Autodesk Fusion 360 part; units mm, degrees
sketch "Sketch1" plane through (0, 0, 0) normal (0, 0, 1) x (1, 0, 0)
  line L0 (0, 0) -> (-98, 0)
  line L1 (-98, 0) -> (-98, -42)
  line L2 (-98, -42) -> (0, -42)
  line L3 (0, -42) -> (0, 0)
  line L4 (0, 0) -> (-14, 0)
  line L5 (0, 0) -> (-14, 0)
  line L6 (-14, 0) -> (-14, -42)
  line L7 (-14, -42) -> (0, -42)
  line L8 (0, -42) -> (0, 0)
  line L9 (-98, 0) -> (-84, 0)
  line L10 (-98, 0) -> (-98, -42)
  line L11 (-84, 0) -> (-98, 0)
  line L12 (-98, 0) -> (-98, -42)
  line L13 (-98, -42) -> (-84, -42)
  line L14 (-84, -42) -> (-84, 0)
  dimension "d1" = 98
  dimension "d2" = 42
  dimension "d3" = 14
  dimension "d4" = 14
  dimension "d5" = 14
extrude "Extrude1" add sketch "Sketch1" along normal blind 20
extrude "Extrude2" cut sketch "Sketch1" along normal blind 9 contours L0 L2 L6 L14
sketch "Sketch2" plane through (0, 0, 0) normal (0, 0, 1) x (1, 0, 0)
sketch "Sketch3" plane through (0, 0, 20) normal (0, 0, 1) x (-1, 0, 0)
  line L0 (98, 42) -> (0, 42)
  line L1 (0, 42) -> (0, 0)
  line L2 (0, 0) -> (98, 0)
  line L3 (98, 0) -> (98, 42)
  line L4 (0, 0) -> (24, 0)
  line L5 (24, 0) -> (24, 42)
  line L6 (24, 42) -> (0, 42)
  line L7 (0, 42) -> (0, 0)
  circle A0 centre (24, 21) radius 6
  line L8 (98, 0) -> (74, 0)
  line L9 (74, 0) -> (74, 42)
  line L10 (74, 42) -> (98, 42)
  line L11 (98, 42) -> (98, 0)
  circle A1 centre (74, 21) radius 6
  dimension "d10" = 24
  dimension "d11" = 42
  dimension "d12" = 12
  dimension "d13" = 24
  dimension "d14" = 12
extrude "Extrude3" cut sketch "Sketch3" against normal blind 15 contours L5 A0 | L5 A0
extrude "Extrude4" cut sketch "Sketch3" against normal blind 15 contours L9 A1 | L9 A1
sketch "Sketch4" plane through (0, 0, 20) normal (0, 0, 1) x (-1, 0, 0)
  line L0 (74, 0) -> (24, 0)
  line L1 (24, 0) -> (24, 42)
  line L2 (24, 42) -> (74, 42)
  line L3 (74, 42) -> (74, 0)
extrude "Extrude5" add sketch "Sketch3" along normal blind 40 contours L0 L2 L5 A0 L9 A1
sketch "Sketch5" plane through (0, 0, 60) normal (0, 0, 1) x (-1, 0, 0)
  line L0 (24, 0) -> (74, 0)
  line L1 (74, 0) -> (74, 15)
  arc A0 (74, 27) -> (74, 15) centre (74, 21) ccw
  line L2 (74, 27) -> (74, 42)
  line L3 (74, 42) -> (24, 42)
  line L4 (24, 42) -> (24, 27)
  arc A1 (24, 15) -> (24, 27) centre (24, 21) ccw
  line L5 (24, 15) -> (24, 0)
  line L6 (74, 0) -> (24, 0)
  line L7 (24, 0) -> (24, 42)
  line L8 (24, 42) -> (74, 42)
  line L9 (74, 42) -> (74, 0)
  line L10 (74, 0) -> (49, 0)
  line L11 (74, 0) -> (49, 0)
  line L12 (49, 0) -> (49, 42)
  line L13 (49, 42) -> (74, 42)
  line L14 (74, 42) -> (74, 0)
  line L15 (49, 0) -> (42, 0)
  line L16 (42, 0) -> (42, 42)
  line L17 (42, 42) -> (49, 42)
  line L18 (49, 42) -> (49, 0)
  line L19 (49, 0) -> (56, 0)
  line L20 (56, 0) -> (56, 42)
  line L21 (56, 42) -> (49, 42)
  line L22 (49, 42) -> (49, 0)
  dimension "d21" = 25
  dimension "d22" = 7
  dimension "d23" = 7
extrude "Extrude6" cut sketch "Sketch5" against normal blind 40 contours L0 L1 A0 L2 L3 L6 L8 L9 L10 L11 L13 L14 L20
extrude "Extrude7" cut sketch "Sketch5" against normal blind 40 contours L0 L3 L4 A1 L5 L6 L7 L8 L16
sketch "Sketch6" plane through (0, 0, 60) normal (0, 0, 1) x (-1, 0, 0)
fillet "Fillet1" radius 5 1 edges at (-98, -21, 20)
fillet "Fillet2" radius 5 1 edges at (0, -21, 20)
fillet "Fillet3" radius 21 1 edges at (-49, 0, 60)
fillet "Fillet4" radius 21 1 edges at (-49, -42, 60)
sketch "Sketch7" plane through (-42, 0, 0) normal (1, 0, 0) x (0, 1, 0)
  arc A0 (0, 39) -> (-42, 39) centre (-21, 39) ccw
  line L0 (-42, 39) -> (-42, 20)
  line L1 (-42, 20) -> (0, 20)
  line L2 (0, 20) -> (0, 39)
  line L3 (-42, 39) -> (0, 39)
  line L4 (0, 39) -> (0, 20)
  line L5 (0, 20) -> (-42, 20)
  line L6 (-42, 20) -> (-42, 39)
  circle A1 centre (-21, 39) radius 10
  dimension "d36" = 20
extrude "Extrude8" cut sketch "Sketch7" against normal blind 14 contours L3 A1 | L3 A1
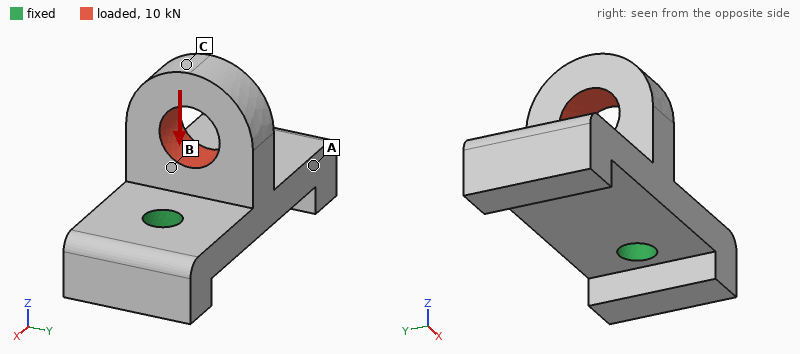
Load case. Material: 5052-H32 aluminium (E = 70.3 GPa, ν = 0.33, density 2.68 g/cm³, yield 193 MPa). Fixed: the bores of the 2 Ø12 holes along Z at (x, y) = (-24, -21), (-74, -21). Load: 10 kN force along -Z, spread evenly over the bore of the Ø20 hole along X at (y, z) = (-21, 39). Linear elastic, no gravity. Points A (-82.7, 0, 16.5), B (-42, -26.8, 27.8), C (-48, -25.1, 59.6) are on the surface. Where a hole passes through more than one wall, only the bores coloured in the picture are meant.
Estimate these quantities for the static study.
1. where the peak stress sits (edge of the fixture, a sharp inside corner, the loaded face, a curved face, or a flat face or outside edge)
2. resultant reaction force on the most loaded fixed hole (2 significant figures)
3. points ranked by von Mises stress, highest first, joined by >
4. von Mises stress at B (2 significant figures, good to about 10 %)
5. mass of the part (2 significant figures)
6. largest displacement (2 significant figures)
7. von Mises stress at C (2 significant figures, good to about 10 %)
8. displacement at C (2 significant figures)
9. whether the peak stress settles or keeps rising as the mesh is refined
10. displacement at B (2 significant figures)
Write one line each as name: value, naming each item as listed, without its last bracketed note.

where the peak stress sits: edge of the fixture
resultant reaction force on the most loaded fixed hole: 5.1 kN
points ranked by von Mises stress, highest first, joined by >: B > C > A
von Mises stress at B: 30 MPa
mass of the part: 190 g
largest displacement: 37 µm
von Mises stress at C: 21 MPa
displacement at C: 35 µm
whether the peak stress settles or keeps rising as the mesh is refined: keeps rising
displacement at B: 21 µm
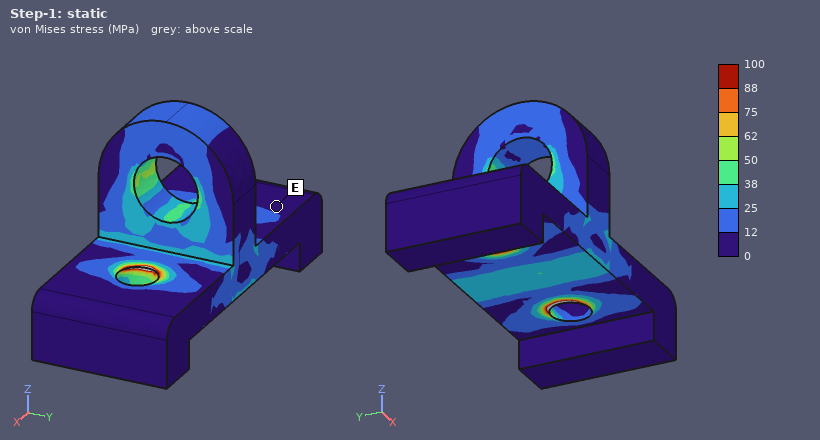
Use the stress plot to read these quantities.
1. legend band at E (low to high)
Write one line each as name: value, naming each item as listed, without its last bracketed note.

legend band at E: 0 to 12 MPa
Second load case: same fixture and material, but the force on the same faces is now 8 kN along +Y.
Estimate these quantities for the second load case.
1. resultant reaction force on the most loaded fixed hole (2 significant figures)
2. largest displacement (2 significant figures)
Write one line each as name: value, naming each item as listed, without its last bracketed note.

resultant reaction force on the most loaded fixed hole: 4.0 kN
largest displacement: 0.18 mm
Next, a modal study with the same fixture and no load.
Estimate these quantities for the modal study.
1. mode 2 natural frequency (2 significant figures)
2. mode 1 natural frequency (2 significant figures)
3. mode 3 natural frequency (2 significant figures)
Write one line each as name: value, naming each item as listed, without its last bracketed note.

mode 2 natural frequency: 5700 Hz
mode 1 natural frequency: 5600 Hz
mode 3 natural frequency: 11 kHz
